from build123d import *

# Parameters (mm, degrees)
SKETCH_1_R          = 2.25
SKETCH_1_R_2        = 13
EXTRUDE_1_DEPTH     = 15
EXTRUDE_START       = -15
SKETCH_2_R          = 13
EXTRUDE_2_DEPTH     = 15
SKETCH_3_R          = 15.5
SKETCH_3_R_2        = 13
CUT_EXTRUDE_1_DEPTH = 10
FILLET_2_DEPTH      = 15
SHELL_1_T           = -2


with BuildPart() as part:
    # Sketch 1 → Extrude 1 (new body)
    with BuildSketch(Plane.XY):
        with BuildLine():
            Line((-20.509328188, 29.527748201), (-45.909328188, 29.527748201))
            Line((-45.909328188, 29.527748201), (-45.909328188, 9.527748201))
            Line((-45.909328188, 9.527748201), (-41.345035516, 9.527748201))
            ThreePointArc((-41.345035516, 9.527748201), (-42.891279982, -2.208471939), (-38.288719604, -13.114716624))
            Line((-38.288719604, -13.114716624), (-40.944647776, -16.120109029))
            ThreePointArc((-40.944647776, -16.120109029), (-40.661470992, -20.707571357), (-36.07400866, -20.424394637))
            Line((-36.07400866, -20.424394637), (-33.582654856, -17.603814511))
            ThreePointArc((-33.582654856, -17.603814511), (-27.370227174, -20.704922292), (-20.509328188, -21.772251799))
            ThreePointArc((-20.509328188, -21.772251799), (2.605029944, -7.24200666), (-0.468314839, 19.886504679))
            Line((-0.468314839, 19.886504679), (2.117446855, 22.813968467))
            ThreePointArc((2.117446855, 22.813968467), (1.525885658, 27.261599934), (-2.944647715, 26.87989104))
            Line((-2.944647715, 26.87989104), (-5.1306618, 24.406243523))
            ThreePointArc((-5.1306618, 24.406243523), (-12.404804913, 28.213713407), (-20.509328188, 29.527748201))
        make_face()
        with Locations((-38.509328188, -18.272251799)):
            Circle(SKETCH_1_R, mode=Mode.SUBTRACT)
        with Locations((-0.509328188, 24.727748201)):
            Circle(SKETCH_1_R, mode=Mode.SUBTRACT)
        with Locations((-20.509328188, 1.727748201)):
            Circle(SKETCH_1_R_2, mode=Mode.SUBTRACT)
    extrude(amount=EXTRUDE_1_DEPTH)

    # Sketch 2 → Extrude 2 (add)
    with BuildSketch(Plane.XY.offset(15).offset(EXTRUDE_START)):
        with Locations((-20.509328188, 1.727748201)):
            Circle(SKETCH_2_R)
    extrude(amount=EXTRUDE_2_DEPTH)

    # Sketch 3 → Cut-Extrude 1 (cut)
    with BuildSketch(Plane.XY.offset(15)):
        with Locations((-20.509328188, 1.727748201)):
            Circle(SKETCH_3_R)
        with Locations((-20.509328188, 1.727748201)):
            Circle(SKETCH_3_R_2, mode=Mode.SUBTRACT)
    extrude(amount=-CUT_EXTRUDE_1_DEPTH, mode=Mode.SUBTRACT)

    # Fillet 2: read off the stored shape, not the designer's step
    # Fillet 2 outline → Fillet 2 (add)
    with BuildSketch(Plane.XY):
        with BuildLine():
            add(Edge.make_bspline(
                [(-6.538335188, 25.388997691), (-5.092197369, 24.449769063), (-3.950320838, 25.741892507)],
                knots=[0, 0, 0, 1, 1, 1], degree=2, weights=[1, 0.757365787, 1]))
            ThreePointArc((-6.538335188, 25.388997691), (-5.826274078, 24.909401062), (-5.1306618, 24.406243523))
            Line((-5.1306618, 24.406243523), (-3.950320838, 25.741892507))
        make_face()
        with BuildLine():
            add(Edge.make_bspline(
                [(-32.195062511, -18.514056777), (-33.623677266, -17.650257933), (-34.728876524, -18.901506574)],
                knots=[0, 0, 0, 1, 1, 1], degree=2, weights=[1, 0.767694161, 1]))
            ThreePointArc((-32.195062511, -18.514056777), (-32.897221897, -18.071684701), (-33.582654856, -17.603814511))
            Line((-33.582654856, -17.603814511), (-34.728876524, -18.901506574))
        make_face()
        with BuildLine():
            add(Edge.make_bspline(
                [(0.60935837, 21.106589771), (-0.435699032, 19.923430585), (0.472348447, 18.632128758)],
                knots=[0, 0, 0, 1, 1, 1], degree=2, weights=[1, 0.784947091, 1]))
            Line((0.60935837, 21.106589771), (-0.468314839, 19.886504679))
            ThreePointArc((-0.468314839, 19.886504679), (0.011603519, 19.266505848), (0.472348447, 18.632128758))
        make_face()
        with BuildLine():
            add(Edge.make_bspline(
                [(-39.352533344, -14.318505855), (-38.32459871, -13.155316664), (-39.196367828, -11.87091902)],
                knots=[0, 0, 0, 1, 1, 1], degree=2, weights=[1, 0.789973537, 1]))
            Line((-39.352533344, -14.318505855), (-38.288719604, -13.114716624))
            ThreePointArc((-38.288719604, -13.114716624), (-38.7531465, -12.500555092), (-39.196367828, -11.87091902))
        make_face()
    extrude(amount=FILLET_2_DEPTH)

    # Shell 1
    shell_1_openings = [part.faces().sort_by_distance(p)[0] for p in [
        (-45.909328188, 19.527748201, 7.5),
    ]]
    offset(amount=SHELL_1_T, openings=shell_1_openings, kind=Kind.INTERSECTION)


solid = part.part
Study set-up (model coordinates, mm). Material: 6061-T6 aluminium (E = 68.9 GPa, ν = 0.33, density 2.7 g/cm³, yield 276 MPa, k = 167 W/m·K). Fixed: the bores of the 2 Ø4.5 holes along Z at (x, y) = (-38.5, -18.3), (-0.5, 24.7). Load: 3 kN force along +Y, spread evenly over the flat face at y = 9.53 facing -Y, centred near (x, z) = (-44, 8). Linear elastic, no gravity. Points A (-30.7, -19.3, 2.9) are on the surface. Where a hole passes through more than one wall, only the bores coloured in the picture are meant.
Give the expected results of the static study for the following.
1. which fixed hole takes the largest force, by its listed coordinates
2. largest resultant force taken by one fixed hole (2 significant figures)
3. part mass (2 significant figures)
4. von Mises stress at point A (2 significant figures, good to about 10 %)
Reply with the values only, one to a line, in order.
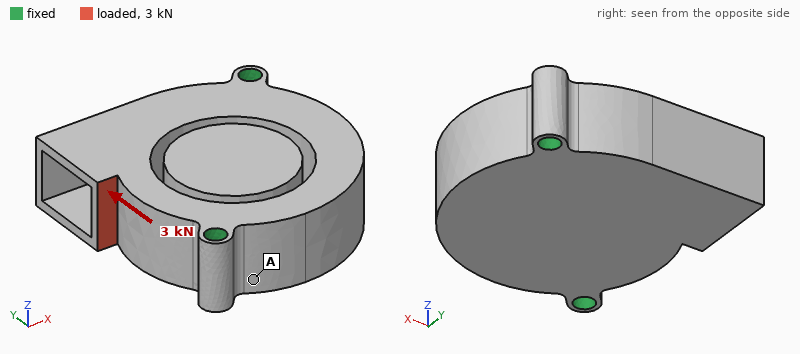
(-38.5, -18.3)
2.8 kN
43 g
23 MPa
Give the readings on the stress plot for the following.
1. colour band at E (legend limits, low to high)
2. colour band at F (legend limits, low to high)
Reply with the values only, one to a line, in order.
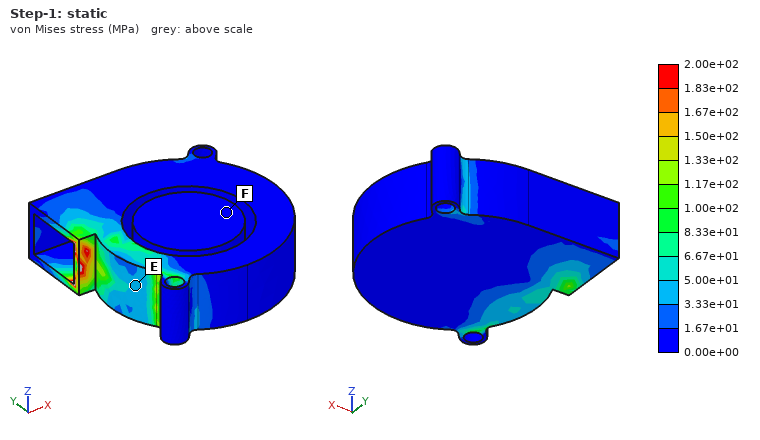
3.33e+01 to 5.00e+01 MPa
0.00e+00 to 1.67e+01 MPa
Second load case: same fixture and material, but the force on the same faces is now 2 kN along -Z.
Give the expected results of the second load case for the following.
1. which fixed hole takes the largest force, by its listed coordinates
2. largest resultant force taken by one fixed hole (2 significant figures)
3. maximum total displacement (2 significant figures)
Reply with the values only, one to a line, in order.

(-38.5, -18.3)
1.7 kN
0.16 mm
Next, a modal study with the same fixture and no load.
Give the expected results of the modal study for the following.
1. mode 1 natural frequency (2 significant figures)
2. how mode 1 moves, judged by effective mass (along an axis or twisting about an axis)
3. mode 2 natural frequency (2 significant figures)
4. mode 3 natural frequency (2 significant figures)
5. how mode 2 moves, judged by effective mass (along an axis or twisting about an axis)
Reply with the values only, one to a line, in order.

6100 Hz
along Z
7000 Hz
8100 Hz
along Z
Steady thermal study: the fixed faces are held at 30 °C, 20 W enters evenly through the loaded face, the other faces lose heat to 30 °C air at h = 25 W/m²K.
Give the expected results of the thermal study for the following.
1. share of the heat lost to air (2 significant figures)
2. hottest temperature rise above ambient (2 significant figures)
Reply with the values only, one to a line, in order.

15 %
36 K
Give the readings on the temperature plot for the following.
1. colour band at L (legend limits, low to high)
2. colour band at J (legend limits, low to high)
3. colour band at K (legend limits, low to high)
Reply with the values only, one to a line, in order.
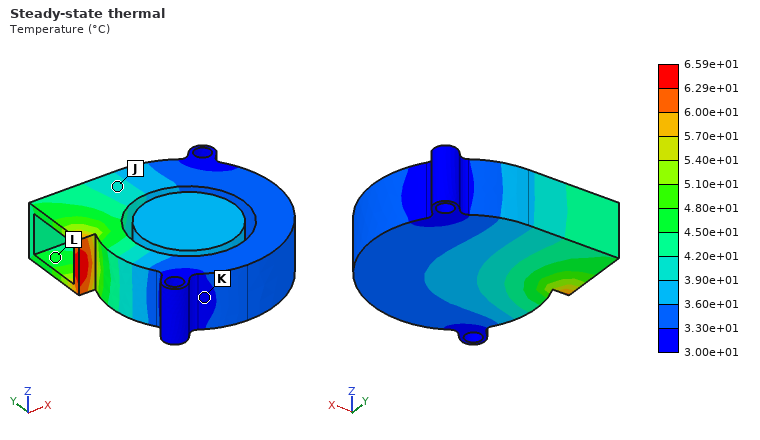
4.50e+01 to 4.80e+01 °C
3.90e+01 to 4.20e+01 °C
3.00e+01 to 3.30e+01 °C
